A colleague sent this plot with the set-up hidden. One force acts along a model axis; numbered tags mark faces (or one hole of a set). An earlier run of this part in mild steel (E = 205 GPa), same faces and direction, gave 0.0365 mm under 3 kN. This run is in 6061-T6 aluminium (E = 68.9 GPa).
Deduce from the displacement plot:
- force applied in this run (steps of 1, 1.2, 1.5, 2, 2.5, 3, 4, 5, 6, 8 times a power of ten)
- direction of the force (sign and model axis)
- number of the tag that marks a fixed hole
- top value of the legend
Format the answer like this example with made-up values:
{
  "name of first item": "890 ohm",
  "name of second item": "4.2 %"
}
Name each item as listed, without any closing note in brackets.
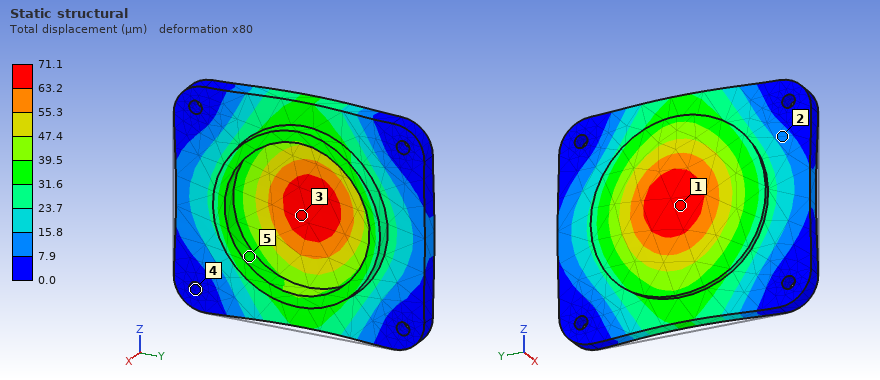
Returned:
{
  "force applied in this run": "2 kN",
  "direction of the force": "-X",
  "number of the tag that marks a fixed hole": "4",
  "top value of the legend": "71.1 µm"
}
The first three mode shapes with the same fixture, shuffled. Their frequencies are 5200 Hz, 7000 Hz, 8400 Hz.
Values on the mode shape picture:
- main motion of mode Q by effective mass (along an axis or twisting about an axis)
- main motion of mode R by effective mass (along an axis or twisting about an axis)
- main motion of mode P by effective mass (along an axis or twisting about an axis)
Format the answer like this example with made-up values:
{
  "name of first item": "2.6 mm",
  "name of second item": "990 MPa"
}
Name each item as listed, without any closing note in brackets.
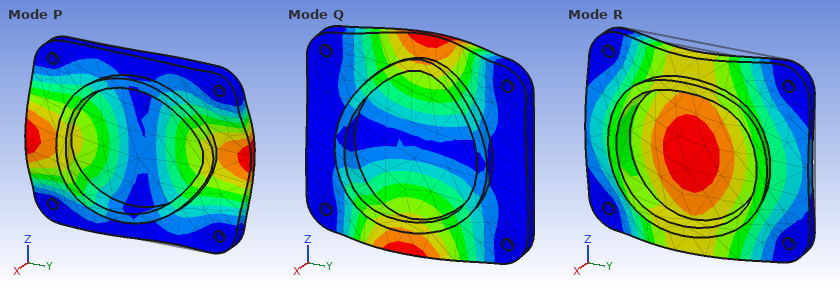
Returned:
{
  "main motion of mode Q by effective mass": "twisting about Y",
  "main motion of mode R by effective mass": "along X",
  "main motion of mode P by effective mass": "twisting about Z"
}
